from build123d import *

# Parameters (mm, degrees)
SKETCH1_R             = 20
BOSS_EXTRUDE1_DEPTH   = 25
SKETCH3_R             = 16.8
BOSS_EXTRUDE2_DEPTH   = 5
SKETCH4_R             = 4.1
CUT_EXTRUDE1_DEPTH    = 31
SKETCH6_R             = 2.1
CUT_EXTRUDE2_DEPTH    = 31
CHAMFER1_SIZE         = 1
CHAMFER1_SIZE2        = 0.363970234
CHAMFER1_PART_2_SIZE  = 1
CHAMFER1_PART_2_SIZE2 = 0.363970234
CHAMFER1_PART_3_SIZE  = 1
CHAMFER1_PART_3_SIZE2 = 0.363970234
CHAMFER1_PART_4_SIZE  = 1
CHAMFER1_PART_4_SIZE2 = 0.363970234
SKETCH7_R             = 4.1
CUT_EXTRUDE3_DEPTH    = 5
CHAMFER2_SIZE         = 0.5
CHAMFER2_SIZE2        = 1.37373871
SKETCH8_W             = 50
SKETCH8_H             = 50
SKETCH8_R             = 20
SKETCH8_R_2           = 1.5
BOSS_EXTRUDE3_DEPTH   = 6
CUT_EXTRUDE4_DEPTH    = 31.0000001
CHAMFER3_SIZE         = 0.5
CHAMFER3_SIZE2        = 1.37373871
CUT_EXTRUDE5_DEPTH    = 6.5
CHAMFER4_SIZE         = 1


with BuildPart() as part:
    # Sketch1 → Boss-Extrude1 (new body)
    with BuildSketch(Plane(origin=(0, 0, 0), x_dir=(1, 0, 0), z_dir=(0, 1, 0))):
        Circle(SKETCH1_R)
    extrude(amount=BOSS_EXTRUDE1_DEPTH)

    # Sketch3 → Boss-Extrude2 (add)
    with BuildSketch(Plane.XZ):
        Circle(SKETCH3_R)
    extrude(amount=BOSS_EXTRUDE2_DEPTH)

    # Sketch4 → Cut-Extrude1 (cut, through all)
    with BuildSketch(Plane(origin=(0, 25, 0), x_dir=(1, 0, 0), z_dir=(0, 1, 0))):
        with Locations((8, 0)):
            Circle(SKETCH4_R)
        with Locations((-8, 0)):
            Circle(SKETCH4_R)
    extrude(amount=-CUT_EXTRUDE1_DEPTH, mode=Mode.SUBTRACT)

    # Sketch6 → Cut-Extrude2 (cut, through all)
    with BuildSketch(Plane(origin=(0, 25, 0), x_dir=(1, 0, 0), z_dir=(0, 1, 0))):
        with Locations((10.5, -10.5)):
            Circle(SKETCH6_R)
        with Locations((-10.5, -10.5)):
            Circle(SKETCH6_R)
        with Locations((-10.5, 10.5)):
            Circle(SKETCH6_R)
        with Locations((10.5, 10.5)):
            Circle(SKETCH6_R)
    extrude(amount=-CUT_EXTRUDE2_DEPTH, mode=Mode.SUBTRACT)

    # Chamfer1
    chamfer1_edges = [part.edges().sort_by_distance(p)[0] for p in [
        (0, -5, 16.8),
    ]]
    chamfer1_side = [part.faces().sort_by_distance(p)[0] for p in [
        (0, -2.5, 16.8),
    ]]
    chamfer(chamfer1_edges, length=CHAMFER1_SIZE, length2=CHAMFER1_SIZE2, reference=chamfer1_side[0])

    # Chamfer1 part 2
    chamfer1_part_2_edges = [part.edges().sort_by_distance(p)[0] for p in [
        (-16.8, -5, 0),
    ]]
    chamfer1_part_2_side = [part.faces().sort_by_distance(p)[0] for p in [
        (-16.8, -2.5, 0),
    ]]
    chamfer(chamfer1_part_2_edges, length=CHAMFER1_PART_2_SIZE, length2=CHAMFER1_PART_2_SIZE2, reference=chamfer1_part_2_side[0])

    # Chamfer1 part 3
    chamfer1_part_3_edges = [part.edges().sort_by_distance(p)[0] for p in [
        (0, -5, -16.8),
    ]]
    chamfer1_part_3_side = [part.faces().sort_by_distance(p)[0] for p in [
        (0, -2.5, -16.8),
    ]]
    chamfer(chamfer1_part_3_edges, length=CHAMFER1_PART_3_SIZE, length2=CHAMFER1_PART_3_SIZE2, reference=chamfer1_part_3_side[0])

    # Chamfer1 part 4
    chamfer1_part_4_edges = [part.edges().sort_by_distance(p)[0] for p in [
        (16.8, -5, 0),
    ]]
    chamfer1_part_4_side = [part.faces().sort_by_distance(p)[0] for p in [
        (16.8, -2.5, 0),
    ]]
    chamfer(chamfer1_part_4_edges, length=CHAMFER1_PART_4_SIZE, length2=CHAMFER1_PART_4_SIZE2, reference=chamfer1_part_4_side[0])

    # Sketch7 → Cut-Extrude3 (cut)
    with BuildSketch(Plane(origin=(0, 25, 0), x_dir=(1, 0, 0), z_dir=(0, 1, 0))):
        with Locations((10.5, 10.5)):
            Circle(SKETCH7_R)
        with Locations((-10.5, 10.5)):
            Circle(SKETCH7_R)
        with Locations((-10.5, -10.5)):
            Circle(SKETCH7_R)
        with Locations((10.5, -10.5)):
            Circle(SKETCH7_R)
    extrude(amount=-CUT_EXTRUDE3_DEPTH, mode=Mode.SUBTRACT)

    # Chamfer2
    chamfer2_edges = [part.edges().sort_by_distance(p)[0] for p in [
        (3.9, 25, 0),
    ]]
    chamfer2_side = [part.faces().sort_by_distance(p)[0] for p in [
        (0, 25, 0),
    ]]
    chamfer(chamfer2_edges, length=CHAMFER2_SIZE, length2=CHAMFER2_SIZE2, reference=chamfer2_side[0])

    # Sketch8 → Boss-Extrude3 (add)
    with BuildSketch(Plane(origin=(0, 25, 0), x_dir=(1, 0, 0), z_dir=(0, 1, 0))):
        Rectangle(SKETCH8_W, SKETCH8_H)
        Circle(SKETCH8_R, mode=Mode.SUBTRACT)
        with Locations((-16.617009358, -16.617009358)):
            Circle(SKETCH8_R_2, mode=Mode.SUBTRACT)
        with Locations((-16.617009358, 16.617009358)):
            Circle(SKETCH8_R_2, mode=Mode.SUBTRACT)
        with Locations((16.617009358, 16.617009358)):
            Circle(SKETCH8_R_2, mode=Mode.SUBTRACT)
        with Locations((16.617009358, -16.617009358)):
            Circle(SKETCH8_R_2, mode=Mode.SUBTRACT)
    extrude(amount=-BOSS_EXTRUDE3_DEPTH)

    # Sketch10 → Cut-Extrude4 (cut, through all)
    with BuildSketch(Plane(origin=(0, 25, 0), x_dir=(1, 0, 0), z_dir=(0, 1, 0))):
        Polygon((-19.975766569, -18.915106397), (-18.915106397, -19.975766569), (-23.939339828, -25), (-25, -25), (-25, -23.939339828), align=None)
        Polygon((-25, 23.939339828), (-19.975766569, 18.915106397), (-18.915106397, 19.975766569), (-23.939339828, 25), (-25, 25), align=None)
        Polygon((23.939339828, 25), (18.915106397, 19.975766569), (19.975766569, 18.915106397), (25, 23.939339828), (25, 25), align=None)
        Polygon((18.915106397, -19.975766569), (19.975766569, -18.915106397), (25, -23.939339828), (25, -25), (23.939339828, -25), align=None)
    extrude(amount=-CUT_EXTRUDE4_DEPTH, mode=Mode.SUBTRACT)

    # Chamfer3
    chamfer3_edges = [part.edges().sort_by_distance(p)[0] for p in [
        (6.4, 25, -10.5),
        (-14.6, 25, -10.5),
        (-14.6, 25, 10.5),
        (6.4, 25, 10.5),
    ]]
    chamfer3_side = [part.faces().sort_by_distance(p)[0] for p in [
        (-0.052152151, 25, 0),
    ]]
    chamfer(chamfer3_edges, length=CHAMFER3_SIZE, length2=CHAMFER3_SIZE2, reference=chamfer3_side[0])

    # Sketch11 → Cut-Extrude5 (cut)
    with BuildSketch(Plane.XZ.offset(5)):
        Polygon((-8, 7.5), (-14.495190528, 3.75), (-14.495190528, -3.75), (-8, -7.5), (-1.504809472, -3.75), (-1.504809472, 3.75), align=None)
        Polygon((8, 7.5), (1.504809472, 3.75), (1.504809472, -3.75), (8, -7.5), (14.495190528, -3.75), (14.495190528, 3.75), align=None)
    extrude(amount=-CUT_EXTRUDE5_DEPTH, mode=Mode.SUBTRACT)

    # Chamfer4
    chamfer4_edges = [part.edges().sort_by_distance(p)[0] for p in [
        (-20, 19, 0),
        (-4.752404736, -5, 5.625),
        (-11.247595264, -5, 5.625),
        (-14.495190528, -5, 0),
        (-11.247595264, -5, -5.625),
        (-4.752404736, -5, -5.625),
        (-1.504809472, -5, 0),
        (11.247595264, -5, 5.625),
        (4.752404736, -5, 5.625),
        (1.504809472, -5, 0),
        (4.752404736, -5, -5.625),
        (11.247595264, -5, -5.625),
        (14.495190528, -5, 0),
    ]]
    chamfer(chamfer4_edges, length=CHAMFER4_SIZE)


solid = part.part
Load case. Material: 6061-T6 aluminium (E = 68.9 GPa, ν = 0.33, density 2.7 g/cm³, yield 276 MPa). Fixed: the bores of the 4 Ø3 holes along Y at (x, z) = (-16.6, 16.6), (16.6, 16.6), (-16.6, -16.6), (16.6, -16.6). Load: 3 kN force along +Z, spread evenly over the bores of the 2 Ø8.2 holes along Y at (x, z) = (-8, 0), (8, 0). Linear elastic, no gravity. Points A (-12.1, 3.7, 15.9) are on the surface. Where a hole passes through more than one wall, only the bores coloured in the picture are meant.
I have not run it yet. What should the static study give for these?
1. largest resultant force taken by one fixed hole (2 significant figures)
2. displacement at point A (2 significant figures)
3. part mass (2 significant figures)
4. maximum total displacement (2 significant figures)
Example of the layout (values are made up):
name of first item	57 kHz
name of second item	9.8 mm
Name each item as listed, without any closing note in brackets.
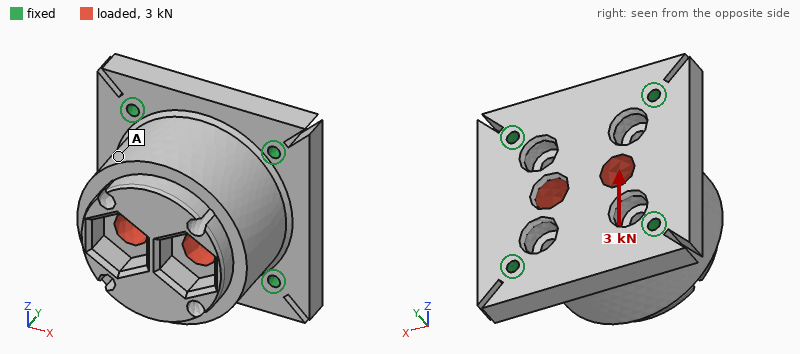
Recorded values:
largest resultant force taken by one fixed hole	870 N
displacement at point A	5.1 µm
part mass	97 g
maximum total displacement	6.2 µm
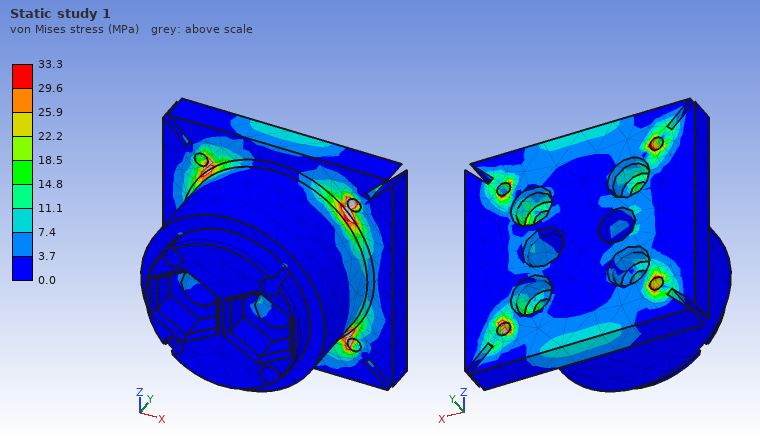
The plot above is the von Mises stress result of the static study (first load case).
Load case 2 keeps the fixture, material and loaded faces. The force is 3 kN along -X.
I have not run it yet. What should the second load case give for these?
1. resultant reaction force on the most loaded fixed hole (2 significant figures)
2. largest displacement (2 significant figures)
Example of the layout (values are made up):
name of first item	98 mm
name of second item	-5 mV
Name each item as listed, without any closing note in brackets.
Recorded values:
resultant reaction force on the most loaded fixed hole	870 N
largest displacement	6.2 µm
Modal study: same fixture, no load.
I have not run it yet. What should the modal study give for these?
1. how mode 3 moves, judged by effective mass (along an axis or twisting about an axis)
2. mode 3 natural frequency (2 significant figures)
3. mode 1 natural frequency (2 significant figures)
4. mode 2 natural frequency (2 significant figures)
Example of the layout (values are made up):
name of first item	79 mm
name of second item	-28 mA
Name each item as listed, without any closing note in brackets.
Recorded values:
how mode 3 moves, judged by effective mass	along Y
mode 3 natural frequency	15 kHz
mode 1 natural frequency	13 kHz
mode 2 natural frequency	13 kHz
